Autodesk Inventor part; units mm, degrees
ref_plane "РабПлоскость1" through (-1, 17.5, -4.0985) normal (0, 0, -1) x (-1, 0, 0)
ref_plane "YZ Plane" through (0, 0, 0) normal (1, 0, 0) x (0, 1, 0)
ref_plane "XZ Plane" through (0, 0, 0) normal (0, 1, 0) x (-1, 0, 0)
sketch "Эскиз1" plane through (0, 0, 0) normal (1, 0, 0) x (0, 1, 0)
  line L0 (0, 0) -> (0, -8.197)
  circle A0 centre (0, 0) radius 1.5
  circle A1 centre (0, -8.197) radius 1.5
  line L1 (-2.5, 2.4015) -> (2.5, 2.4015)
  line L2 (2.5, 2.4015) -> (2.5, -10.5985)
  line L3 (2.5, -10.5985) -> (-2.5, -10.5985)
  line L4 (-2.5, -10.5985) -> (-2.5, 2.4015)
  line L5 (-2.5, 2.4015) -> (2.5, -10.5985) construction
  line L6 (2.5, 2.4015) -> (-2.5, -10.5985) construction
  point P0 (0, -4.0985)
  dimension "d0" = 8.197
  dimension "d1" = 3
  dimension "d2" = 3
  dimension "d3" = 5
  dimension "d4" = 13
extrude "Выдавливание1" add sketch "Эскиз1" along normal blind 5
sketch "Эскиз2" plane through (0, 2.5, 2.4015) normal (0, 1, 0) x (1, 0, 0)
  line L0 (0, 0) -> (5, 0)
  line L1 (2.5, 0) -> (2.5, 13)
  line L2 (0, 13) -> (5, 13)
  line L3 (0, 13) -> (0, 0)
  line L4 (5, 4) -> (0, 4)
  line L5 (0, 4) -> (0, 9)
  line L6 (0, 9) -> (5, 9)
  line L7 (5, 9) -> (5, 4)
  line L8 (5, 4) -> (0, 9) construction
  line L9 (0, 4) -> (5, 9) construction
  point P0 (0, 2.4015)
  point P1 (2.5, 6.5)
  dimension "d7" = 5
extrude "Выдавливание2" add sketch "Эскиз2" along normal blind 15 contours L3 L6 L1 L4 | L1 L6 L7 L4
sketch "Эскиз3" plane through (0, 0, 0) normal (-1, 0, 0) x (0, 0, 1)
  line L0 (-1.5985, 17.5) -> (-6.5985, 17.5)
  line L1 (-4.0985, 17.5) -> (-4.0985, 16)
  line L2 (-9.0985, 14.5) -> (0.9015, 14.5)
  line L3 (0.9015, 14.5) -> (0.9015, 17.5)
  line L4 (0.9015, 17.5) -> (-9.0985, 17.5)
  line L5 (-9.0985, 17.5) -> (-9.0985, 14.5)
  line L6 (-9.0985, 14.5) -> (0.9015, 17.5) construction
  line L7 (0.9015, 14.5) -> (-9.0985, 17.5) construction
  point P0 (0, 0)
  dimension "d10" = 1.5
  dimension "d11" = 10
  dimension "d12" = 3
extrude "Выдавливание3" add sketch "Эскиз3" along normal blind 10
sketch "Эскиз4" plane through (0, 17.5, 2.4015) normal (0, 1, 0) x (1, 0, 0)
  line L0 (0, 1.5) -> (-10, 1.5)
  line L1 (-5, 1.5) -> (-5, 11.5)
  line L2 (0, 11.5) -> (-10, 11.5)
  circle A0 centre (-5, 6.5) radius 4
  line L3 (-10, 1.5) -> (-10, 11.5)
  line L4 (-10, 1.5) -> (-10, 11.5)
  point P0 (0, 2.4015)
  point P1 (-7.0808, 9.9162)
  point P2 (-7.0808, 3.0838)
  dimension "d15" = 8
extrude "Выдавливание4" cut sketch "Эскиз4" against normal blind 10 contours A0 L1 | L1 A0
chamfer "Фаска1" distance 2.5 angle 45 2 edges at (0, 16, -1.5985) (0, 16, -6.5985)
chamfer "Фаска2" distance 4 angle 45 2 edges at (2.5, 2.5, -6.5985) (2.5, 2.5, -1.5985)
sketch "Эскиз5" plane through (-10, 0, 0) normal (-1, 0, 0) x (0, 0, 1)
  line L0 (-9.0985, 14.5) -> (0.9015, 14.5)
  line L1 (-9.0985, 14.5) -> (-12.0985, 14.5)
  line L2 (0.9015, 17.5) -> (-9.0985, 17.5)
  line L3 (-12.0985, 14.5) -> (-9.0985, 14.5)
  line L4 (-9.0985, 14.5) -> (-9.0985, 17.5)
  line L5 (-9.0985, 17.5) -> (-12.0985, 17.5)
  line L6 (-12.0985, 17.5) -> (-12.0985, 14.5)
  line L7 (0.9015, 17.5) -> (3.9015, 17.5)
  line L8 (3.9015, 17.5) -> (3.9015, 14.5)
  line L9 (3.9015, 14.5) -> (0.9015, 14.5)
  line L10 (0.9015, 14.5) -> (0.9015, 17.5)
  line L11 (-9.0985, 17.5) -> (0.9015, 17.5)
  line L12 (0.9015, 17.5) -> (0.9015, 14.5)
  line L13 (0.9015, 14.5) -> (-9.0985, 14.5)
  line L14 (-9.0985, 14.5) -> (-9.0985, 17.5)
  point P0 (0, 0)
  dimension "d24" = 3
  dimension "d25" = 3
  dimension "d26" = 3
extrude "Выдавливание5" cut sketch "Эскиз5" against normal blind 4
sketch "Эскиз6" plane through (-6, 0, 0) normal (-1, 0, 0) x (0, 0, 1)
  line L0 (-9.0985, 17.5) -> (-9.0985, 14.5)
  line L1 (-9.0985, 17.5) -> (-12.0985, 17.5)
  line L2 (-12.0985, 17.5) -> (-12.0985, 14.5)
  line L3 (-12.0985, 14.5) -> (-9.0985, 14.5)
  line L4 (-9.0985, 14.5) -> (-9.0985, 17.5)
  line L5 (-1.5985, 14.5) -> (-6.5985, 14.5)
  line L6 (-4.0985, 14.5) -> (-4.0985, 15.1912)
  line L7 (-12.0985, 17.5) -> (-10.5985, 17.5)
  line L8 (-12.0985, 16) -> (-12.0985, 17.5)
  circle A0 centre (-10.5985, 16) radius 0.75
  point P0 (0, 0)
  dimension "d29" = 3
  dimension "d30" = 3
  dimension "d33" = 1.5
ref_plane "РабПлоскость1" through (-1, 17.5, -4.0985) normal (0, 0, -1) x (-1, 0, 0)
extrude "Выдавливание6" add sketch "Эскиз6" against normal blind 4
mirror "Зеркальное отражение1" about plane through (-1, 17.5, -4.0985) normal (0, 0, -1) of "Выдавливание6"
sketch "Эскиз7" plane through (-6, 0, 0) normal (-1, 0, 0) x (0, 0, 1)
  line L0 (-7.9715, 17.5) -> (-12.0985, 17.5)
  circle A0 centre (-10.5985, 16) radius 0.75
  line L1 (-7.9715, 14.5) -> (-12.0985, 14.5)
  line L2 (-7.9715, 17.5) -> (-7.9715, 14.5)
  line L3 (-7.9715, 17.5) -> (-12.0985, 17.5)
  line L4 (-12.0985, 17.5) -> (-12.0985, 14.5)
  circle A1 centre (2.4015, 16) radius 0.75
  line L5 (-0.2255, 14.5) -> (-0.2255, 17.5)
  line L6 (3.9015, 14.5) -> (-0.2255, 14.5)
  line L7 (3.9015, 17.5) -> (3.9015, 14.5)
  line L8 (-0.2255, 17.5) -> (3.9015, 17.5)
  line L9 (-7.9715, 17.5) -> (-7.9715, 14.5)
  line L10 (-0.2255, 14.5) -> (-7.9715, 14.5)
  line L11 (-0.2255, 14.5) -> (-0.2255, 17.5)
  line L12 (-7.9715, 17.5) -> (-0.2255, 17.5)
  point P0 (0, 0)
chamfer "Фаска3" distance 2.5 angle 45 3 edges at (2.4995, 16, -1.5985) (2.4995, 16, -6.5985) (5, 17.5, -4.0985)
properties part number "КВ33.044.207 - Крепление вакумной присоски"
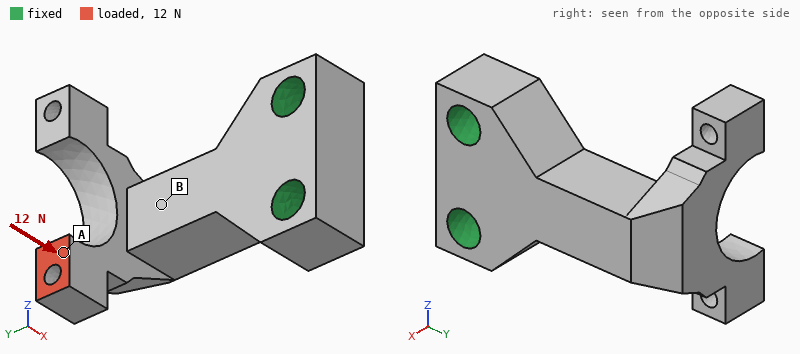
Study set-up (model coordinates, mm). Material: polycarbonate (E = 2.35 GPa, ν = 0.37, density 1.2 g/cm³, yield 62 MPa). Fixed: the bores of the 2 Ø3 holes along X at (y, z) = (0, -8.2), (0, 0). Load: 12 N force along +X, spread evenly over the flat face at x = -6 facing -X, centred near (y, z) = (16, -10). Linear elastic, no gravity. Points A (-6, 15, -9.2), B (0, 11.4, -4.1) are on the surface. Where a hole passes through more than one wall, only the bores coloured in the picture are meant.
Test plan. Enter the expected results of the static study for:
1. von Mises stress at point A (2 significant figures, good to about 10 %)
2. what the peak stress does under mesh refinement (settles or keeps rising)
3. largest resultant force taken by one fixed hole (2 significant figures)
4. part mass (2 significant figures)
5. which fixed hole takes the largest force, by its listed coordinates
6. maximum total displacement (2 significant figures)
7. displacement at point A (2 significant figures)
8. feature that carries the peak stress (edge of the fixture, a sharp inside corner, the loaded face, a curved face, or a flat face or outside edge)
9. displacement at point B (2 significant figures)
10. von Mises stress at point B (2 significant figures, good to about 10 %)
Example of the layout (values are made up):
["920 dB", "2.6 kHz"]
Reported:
["1.5 MPa", "keeps rising", "13 N", "1.0 g", "(0, -8.2)", "0.31 mm", "0.24 mm", "a sharp inside corner", "0.057 mm", "5.5 MPa"]
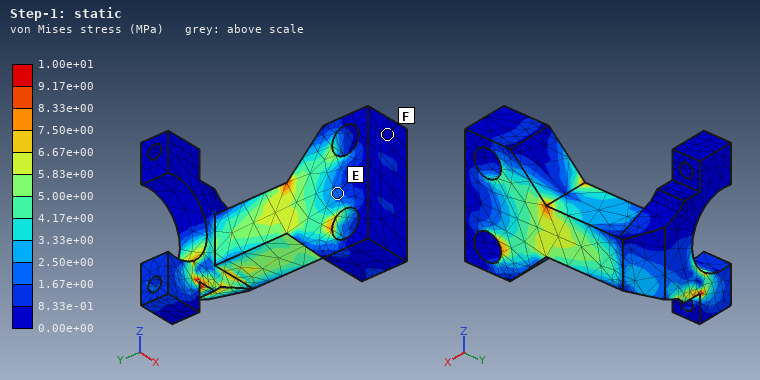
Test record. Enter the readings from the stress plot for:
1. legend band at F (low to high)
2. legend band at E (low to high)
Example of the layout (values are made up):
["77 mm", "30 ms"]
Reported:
["0.00e+00 to 8.33e-01 MPa", "1.67e+00 to 2.50e+00 MPa"]
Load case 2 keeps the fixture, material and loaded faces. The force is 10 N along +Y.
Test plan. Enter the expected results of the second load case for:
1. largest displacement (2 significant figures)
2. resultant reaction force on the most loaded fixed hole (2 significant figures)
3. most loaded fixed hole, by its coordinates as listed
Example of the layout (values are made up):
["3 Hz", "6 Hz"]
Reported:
["0.31 mm", "12 N", "(0, -8.2)"]
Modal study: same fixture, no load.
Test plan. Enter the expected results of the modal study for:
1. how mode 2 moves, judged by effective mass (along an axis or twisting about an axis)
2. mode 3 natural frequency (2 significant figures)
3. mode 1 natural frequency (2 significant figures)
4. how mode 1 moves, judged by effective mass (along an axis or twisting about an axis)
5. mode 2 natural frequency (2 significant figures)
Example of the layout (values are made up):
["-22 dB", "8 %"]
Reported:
["along Z", "4700 Hz", "2800 Hz", "along X", "3100 Hz"]
